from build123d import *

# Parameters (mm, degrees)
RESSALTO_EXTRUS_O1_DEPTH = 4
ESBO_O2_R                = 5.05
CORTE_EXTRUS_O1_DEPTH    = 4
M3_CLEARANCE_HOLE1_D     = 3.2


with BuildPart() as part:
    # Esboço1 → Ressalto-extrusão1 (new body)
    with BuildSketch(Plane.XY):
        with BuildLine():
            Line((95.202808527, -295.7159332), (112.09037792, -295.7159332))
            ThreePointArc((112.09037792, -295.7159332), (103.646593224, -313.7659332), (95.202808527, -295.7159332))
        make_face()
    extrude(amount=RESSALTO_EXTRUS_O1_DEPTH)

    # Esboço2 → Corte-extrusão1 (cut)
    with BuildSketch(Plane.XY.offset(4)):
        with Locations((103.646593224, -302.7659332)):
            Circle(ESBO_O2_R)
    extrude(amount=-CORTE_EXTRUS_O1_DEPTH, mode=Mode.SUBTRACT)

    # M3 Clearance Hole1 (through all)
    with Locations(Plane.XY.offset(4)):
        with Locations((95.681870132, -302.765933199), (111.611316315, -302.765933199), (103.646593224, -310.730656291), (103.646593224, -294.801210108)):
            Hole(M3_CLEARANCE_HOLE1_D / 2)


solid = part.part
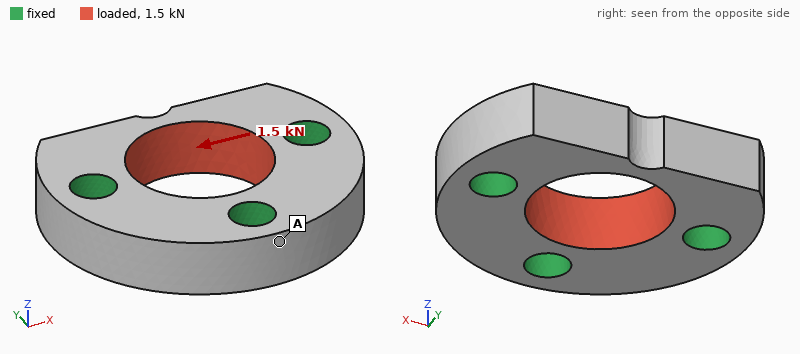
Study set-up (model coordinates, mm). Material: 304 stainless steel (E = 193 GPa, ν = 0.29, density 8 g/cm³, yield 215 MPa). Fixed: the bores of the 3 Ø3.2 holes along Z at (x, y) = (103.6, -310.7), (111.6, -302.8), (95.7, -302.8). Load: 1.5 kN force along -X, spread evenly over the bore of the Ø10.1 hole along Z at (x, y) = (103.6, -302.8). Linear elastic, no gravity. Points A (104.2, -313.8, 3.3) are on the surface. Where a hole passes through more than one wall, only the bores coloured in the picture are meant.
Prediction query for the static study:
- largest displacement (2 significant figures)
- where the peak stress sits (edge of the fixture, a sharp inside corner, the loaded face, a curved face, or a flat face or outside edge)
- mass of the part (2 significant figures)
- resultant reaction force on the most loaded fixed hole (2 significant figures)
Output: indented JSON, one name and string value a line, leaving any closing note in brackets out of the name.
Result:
{
  "largest displacement": "1.7 µm",
  "where the peak stress sits": "edge of the fixture",
  "mass of the part": "7.3 g",
  "resultant reaction force on the most loaded fixed hole": "570 N"
}
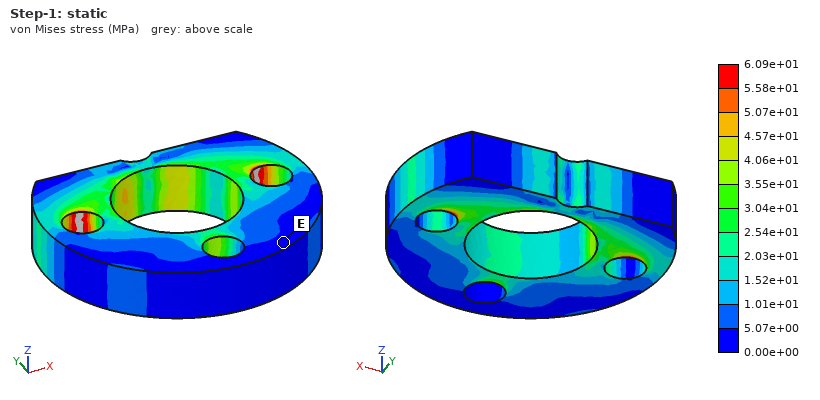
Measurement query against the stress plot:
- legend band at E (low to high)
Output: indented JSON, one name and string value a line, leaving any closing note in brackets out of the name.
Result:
{
  "legend band at E": "0.00e+00 to 5.07e+00 MPa"
}
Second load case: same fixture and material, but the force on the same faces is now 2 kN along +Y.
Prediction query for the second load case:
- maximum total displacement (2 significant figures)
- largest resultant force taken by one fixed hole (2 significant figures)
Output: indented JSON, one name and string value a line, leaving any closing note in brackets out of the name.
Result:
{
  "maximum total displacement": "4.3 µm",
  "largest resultant force taken by one fixed hole": "780 N"
}
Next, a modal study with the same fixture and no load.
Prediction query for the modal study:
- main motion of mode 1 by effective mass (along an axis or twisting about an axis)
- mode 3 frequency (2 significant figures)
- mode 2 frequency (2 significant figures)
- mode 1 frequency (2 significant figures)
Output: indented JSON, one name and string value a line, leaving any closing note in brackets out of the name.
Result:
{
  "main motion of mode 1 by effective mass": "along Z",
  "mode 3 frequency": "72 kHz",
  "mode 2 frequency": "70 kHz",
  "mode 1 frequency": "48 kHz"
}
